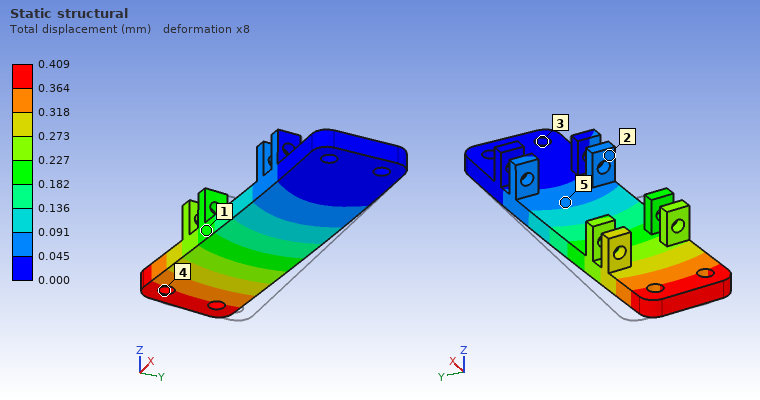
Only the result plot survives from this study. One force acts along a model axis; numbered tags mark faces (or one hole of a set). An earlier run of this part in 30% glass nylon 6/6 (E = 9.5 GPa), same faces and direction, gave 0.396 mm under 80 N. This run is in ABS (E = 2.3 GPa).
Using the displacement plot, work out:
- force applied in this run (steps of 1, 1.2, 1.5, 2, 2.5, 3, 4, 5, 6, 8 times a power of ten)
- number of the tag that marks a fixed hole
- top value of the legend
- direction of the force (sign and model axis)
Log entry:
20 N
3
0.409 mm
-Y
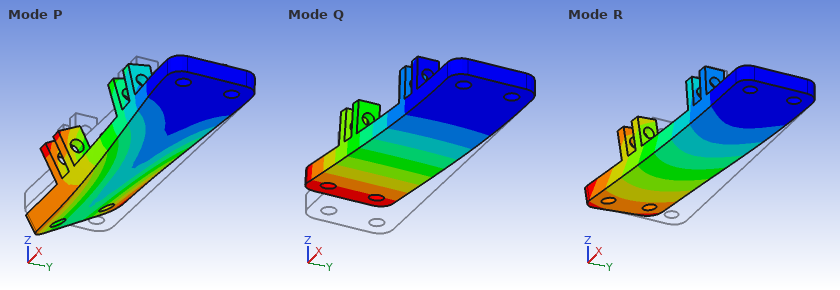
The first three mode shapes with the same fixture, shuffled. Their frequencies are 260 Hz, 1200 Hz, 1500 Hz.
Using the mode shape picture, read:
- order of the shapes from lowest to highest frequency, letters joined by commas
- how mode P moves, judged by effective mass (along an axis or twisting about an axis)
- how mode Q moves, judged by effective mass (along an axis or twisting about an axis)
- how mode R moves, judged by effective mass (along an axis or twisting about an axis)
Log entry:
Q, R, P
twisting about X
along Z
along Y
